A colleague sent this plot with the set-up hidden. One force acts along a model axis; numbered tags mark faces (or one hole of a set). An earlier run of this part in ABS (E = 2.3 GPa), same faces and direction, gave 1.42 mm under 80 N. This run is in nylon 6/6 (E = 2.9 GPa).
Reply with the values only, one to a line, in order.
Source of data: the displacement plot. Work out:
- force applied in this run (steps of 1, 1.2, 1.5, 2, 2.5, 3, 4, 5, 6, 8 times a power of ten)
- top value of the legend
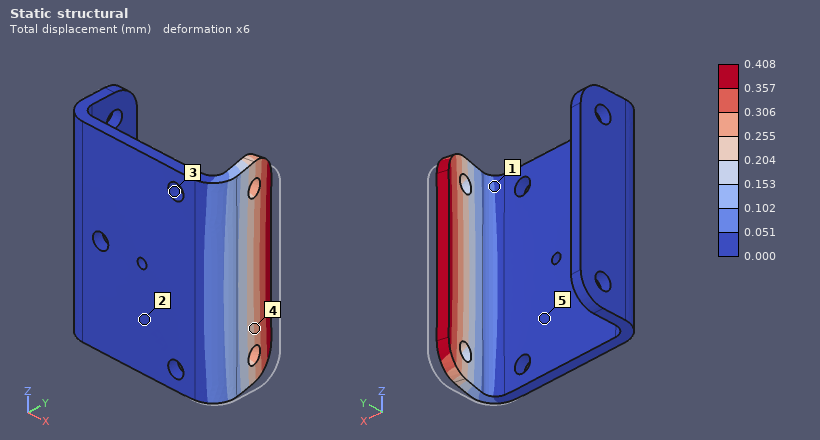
30 N
0.408 mm
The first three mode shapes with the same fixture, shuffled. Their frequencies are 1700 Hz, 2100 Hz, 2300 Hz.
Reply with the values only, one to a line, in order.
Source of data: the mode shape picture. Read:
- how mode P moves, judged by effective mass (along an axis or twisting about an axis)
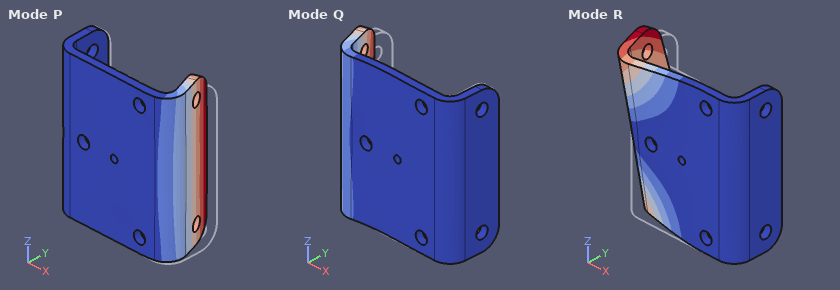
along X
